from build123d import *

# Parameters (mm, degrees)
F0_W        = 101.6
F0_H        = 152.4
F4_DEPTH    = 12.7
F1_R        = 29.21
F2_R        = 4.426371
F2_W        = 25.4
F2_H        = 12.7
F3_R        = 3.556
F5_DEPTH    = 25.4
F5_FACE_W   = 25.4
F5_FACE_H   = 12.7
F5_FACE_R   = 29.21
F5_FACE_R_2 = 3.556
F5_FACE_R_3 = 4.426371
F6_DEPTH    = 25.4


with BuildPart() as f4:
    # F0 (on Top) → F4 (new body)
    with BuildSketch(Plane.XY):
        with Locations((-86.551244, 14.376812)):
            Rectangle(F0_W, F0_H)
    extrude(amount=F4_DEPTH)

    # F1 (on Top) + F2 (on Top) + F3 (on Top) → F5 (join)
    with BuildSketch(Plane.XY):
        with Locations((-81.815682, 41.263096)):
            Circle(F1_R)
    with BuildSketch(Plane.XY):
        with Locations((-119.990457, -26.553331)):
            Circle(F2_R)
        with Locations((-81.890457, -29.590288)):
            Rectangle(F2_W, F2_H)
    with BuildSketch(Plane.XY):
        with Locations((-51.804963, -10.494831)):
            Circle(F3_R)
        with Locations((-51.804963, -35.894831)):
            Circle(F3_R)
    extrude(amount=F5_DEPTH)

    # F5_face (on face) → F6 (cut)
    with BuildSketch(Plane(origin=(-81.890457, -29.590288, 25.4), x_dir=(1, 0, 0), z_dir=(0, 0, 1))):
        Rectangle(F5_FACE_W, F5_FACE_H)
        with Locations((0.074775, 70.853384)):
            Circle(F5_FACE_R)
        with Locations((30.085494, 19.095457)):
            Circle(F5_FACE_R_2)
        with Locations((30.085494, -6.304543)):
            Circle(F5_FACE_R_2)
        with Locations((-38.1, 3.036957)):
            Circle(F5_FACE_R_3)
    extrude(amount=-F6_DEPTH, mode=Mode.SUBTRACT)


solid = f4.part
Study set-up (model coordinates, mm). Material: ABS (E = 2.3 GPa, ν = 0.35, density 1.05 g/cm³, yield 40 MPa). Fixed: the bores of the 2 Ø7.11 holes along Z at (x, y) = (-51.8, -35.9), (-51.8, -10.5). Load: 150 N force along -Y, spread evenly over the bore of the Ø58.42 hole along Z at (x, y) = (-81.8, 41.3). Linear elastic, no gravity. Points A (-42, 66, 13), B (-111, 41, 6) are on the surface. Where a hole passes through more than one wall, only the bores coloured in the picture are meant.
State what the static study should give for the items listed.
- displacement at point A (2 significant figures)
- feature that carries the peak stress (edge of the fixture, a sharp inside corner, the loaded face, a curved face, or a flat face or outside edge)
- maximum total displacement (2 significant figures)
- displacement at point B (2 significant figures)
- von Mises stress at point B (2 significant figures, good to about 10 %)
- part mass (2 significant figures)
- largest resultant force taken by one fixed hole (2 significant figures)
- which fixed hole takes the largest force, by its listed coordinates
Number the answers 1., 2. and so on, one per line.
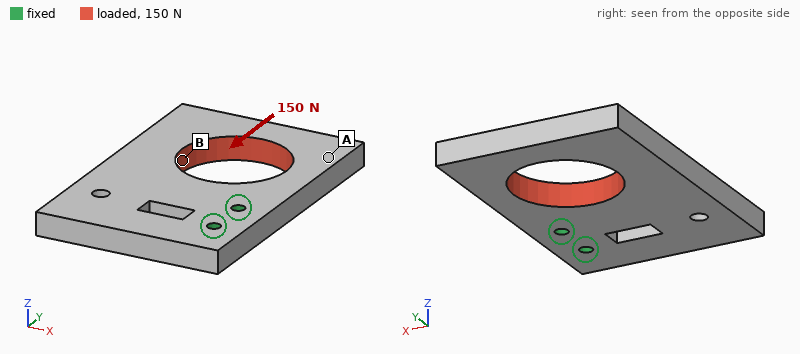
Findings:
1. 35 µm
2. edge of the fixture
3. 65 µm
4. 47 µm
5. 0.38 MPa
6. 160 g
7. 170 N
8. (-51.8, -10.5)
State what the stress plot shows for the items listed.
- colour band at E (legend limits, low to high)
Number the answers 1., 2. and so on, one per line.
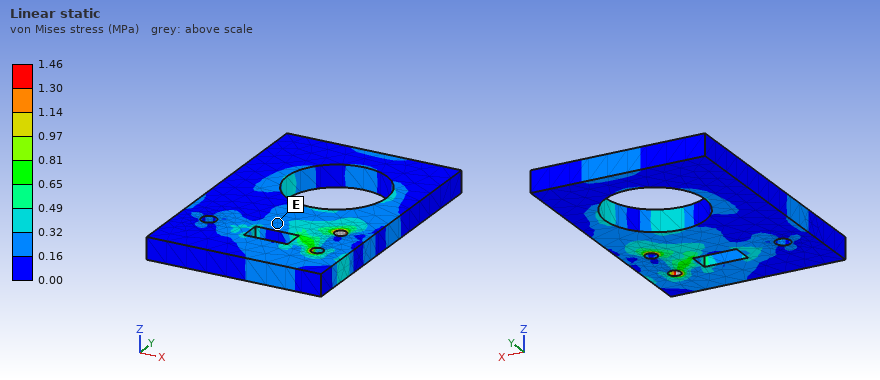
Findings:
1. 0.16 to 0.32 MPa
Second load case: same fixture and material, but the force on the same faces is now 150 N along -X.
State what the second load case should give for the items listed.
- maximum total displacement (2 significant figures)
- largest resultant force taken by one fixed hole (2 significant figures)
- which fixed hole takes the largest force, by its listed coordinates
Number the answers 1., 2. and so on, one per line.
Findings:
1. 0.17 mm
2. 380 N
3. (-51.8, -10.5)
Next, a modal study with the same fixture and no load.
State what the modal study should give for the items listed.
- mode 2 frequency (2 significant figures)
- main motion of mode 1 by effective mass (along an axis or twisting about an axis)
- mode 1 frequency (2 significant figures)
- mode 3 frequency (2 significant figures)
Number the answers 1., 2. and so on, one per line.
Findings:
1. 330 Hz
2. along Z
3. 190 Hz
4. 500 Hz
